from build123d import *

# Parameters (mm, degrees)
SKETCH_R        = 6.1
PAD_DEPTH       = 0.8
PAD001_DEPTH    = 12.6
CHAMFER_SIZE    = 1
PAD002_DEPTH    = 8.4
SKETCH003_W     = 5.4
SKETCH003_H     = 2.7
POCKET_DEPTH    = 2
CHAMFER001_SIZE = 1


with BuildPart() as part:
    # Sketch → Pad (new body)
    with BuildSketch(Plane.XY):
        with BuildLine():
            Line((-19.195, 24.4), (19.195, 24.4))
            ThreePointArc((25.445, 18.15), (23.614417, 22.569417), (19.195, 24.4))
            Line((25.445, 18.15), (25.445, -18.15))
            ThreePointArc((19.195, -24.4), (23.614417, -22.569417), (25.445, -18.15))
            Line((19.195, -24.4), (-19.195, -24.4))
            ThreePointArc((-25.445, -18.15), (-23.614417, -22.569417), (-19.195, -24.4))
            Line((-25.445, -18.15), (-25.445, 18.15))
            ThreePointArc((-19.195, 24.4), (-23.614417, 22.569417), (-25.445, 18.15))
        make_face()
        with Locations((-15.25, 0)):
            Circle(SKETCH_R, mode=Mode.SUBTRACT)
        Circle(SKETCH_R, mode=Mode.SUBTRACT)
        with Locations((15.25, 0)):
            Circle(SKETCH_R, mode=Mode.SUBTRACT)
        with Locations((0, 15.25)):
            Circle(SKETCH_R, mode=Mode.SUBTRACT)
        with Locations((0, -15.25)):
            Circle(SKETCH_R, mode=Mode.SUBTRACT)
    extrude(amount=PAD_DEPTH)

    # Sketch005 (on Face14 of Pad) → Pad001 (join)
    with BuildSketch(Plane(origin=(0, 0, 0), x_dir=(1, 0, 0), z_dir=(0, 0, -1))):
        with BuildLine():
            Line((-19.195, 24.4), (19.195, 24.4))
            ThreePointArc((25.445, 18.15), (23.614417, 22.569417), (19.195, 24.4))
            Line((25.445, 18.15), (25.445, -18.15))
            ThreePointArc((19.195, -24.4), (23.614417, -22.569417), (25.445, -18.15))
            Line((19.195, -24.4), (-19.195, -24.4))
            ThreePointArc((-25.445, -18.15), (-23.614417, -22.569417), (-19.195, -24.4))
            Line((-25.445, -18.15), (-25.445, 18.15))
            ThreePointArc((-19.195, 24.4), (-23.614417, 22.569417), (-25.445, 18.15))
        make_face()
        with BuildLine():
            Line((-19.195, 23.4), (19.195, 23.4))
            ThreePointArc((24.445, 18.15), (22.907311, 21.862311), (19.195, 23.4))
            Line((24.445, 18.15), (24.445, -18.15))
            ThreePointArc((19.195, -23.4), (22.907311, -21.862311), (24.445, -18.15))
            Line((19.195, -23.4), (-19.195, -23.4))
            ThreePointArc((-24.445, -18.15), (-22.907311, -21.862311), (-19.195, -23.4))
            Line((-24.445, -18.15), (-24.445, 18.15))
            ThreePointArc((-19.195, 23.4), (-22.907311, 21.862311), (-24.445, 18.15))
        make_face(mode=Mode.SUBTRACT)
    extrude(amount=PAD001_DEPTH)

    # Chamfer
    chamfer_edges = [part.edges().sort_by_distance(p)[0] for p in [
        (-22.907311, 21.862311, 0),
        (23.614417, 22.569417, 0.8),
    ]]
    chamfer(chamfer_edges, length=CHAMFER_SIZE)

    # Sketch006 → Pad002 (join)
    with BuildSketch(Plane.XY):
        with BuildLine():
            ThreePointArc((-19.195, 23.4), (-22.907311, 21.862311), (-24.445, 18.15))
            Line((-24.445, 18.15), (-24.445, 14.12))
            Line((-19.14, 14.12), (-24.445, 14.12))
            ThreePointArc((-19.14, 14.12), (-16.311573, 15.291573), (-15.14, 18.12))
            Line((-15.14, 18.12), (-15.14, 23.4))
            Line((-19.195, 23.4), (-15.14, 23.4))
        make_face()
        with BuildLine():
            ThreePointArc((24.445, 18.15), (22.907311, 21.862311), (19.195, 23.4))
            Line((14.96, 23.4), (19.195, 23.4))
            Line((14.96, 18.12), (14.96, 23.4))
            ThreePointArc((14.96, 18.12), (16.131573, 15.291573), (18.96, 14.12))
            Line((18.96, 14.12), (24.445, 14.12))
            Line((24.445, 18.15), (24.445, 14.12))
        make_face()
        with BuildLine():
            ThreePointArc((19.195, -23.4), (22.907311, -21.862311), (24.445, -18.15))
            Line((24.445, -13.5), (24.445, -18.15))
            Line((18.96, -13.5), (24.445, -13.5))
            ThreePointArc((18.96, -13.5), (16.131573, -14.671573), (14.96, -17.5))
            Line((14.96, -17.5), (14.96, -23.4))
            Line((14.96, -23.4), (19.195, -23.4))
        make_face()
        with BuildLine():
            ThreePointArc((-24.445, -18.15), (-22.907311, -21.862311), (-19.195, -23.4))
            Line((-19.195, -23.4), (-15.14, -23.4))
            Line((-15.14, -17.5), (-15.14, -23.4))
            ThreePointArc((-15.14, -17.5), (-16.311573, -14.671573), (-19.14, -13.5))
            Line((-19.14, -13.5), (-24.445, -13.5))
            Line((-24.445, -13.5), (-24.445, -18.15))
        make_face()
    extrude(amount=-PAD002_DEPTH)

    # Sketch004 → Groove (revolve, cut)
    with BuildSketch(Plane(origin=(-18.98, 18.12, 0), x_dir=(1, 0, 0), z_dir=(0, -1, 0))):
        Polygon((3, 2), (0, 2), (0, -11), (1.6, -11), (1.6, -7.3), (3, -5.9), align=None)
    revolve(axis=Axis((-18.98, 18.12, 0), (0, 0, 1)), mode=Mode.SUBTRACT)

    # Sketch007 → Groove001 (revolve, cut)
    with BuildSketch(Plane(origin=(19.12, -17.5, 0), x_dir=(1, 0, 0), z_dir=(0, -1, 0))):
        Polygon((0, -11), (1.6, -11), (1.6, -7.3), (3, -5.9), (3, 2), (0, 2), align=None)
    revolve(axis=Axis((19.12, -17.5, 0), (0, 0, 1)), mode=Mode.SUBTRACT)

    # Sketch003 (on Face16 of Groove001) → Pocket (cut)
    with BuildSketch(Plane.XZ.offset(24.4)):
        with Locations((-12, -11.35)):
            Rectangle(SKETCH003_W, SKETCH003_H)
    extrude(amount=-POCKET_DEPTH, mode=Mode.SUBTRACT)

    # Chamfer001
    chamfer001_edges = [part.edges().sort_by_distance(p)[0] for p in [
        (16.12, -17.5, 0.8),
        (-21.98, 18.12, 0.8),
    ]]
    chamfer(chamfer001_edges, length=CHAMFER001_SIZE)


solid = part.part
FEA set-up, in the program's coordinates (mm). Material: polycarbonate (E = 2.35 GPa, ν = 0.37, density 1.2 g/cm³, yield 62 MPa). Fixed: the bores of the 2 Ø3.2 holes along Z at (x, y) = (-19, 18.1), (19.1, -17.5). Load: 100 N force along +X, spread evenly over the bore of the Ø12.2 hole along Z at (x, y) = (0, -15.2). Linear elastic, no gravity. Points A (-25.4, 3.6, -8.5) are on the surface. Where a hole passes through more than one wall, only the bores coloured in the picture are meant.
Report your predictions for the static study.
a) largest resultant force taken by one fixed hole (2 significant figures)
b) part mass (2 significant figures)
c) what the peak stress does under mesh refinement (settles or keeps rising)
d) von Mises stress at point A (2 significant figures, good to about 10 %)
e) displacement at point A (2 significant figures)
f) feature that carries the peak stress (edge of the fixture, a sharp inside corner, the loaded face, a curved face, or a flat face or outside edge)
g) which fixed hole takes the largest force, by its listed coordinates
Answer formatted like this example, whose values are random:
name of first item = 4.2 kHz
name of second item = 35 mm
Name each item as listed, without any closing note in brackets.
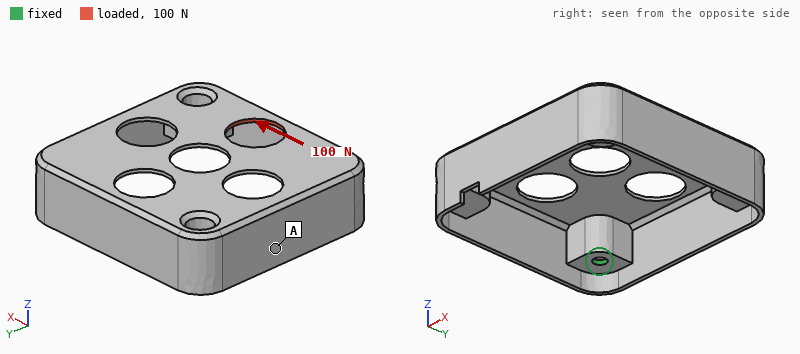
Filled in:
largest resultant force taken by one fixed hole = 76 N
part mass = 7.2 g
what the peak stress does under mesh refinement = keeps rising
von Mises stress at point A = 2.3 MPa
displacement at point A = 0.27 mm
feature that carries the peak stress = edge of the fixture
which fixed hole takes the largest force, by its listed coordinates = (19.1, -17.5)
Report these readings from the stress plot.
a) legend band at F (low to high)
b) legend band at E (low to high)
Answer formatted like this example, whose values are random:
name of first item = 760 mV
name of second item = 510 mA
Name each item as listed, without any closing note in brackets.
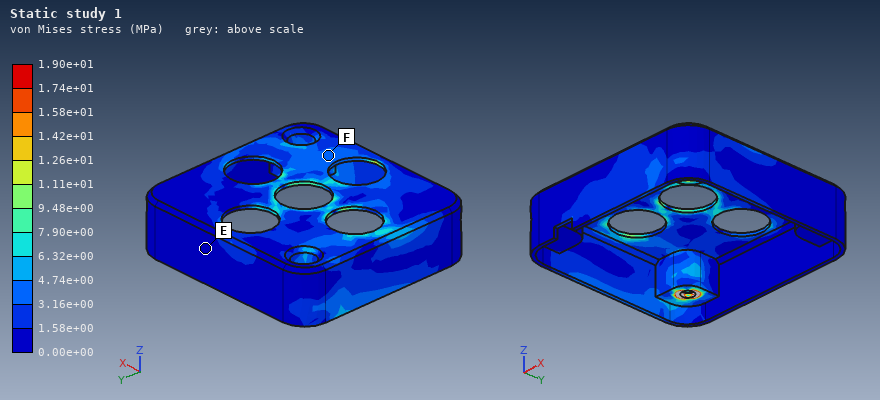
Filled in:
legend band at F = 3.16e+00 to 4.74e+00 MPa
legend band at E = 0.00e+00 to 1.58e+00 MPa
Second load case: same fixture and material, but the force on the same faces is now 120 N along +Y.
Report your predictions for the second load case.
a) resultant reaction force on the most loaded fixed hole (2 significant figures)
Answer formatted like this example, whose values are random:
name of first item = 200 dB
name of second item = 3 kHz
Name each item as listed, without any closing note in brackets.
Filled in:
resultant reaction force on the most loaded fixed hole = 62 N
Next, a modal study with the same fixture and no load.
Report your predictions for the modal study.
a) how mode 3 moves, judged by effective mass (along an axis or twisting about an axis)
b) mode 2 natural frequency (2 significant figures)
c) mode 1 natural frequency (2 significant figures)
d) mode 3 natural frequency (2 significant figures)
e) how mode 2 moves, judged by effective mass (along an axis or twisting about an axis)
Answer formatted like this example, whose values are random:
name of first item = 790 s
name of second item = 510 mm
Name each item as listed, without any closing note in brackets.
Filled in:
how mode 3 moves, judged by effective mass = along Z
mode 2 natural frequency = 920 Hz
mode 1 natural frequency = 500 Hz
mode 3 natural frequency = 1100 Hz
how mode 2 moves, judged by effective mass = along Z
